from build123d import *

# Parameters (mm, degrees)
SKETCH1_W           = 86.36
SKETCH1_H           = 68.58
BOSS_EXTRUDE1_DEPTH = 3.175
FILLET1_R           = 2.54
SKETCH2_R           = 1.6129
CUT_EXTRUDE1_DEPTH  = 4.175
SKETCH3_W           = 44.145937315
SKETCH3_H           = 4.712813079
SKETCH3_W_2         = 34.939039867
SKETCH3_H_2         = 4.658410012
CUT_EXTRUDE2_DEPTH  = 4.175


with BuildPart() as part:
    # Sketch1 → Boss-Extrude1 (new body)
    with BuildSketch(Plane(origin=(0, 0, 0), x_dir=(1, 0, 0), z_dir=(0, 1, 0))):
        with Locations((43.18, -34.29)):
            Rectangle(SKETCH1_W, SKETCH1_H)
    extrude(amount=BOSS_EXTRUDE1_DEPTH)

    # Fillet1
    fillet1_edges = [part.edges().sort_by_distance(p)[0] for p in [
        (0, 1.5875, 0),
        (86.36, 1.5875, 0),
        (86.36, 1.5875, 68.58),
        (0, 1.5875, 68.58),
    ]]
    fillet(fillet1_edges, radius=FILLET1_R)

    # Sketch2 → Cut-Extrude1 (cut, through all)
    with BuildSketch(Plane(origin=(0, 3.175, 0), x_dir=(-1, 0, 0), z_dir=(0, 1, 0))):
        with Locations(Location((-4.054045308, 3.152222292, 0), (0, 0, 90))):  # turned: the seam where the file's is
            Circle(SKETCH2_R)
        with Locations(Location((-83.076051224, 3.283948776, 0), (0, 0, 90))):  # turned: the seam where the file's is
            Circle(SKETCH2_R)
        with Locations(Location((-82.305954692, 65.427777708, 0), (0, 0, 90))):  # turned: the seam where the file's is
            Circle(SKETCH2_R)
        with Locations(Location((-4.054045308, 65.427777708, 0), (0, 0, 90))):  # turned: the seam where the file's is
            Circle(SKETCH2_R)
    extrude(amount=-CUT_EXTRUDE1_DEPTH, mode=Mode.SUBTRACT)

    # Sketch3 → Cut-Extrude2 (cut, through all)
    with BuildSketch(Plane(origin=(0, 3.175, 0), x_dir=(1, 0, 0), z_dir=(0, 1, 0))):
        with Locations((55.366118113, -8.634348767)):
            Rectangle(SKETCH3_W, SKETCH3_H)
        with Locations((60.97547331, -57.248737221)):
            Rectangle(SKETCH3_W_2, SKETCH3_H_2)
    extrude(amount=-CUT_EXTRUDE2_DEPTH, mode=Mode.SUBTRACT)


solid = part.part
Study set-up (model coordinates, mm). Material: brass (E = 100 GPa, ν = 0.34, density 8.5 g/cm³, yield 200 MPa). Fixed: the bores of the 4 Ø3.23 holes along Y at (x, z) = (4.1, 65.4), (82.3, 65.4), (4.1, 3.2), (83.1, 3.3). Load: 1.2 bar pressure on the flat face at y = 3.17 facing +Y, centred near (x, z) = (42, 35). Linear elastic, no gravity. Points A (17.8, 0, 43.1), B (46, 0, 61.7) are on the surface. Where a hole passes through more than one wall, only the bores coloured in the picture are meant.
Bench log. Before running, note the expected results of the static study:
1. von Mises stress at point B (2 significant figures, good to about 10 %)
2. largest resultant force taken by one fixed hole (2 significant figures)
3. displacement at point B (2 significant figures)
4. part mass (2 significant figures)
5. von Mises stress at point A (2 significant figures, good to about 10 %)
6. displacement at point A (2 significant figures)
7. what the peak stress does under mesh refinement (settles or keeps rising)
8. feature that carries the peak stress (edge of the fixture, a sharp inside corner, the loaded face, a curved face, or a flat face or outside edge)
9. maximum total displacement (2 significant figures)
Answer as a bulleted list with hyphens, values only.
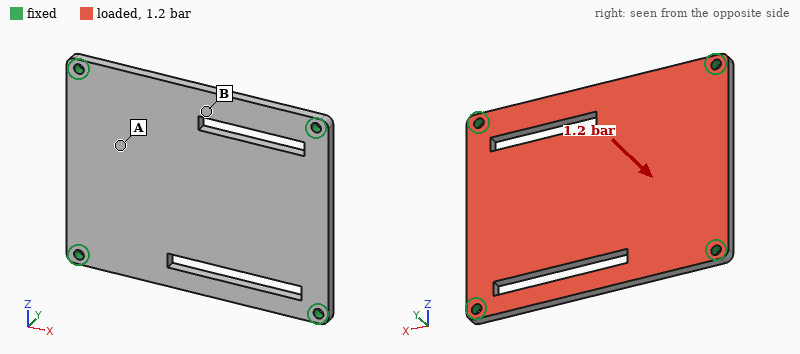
- 36 MPa
- 170 N
- 78 µm
- 150 g
- 14 MPa
- 57 µm
- keeps rising
- edge of the fixture
- 99 µm
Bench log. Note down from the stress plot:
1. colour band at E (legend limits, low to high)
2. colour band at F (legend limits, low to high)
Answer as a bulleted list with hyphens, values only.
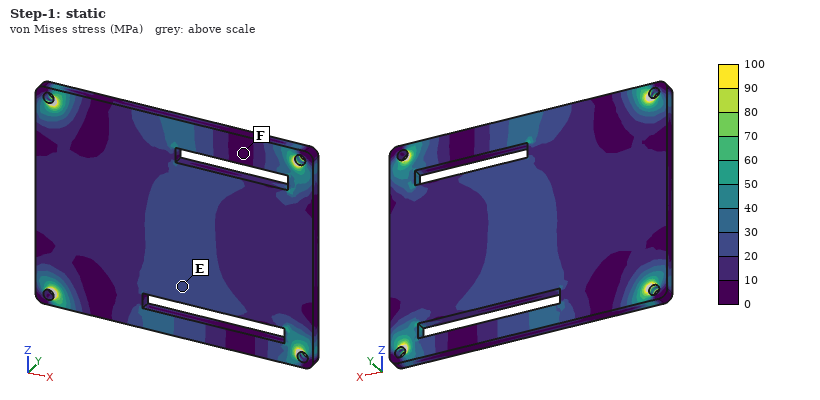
- 20 to 30 MPa
- 0 to 10 MPa
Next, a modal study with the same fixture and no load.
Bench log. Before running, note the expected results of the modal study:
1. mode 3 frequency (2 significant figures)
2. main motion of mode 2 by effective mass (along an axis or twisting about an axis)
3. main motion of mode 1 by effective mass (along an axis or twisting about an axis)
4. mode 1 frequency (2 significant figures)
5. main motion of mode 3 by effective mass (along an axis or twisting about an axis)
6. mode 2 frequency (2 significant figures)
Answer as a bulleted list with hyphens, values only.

- 2600 Hz
- twisting about X
- along Y
- 1200 Hz
- twisting about Z
- 2200 Hz
